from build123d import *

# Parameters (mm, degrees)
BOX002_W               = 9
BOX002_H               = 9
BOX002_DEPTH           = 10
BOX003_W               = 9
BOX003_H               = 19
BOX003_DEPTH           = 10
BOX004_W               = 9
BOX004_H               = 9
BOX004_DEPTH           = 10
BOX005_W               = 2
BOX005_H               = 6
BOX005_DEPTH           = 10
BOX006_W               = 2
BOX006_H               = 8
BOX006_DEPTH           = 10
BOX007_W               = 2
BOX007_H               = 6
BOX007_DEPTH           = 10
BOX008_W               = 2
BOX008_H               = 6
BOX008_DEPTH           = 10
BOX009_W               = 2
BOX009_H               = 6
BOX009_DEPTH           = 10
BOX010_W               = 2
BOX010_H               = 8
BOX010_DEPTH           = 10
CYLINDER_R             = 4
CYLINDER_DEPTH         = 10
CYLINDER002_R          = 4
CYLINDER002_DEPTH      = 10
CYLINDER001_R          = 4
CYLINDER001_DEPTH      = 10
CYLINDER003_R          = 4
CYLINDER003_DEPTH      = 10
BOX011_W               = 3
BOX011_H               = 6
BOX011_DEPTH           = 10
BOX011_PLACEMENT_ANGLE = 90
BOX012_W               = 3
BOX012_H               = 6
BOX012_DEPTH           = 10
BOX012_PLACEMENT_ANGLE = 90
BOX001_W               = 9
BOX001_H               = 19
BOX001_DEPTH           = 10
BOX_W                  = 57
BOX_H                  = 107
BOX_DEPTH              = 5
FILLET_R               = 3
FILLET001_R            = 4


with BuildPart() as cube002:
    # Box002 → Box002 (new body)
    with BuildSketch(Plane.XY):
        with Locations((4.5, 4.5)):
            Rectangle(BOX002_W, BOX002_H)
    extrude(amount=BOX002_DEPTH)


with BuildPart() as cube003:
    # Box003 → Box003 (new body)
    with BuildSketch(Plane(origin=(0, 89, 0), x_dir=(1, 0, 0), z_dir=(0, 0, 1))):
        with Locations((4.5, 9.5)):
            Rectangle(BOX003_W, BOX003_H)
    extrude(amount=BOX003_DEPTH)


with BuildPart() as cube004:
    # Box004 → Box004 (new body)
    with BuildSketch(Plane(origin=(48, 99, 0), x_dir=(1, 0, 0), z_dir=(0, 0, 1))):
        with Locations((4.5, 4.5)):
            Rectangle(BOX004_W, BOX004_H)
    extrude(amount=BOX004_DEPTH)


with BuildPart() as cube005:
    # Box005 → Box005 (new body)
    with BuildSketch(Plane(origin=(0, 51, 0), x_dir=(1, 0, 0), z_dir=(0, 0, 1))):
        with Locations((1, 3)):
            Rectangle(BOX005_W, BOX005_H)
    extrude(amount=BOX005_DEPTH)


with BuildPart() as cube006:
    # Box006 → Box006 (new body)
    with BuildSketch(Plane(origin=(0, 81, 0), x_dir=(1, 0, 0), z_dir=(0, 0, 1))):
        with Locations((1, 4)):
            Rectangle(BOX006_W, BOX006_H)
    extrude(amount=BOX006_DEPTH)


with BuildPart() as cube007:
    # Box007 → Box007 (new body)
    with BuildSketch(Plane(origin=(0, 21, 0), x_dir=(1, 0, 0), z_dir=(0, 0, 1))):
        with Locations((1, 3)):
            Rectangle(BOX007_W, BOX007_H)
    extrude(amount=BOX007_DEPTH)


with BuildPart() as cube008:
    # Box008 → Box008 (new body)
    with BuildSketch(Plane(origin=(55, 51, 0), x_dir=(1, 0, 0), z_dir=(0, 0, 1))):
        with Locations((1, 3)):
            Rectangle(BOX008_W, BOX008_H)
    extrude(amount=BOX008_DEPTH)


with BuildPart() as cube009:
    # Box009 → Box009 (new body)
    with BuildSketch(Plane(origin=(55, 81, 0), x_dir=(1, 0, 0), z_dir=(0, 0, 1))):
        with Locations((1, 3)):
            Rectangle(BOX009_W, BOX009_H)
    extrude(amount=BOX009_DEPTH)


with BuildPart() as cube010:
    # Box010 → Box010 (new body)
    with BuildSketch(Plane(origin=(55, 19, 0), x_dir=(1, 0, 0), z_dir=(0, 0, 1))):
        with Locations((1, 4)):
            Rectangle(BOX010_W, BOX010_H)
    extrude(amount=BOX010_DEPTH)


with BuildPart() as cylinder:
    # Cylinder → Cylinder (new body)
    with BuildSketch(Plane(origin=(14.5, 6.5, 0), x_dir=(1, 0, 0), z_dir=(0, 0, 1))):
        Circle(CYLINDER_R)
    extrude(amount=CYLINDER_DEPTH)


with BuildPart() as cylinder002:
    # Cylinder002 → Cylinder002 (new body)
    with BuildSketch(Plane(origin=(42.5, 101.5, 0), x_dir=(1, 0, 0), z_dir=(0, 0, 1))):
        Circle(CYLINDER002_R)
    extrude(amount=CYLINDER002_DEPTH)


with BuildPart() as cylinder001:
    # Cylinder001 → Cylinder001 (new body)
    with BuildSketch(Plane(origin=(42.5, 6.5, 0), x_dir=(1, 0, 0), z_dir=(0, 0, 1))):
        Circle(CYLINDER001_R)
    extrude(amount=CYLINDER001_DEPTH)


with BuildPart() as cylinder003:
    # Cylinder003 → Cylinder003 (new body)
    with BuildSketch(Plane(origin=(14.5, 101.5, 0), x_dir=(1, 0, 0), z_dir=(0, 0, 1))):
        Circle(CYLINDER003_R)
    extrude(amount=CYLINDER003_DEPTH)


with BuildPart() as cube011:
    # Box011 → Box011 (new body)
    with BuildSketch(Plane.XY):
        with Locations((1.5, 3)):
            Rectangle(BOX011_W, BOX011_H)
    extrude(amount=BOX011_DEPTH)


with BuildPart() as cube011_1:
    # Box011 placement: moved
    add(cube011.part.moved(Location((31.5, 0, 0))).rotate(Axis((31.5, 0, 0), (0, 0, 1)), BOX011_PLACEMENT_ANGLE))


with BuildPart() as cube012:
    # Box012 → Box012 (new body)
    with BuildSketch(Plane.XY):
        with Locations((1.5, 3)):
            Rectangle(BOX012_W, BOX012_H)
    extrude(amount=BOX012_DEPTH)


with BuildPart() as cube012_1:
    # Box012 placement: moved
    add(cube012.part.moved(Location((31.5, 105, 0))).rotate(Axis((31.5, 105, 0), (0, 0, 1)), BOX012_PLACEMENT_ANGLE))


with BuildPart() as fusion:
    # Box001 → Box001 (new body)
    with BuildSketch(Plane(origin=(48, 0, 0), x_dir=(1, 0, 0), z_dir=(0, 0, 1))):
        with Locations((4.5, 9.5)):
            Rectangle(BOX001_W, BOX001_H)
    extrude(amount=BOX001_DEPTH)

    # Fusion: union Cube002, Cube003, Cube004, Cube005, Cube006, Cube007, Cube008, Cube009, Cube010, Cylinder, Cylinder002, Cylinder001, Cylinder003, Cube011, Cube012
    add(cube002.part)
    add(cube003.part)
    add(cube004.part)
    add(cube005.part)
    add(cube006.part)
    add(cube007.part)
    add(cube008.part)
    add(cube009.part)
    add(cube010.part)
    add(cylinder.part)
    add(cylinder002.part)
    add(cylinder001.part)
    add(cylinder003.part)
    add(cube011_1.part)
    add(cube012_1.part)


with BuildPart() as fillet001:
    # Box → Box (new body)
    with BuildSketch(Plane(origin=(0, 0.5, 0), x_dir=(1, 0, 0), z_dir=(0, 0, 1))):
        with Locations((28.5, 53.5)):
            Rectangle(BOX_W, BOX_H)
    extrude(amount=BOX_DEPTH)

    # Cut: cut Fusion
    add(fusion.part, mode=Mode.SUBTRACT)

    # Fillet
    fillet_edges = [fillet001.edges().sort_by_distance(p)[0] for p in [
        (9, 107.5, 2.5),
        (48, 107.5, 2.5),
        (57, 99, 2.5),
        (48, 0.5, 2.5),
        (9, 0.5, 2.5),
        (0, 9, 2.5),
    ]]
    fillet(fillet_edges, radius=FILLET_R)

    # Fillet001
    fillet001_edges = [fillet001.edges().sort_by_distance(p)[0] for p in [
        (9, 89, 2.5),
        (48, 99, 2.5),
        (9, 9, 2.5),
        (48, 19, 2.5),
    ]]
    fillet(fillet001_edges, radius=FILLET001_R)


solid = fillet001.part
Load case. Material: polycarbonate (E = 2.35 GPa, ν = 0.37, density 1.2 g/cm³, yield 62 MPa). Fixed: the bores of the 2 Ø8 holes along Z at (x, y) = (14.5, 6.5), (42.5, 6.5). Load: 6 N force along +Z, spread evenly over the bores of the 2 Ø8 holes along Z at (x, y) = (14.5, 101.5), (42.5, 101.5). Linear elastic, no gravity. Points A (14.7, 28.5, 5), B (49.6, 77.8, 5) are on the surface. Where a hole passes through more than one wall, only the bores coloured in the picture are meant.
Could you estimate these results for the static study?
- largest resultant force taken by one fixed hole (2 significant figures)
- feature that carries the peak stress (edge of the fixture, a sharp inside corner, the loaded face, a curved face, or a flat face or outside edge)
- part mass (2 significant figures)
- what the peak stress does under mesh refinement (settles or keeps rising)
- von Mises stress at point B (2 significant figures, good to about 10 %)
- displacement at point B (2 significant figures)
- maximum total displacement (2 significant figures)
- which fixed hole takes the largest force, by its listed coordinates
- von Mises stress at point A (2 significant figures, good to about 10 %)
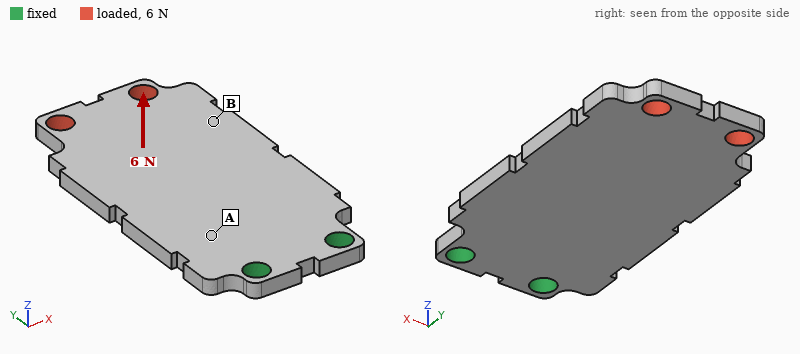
3.8 N
edge of the fixture
32 g
keeps rising
0.64 MPa
0.80 mm
1.4 mm
(14.5, 6.5)
1.9 MPa
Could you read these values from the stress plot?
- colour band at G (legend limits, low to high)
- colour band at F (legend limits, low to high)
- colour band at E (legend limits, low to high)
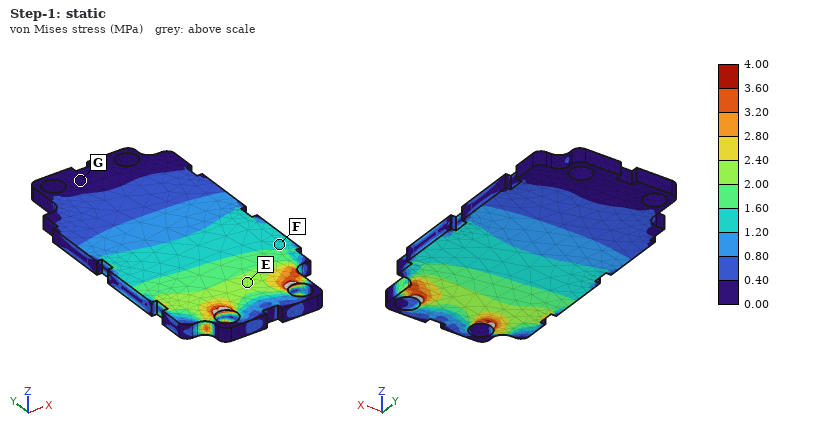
0.00 to 0.40 MPa
1.20 to 1.60 MPa
2.00 to 2.40 MPa
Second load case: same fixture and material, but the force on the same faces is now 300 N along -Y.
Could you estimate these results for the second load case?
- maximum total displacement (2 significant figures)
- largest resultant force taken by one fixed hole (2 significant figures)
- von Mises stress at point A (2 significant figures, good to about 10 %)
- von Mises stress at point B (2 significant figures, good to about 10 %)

83 µm
150 N
1.2 MPa
1.1 MPa
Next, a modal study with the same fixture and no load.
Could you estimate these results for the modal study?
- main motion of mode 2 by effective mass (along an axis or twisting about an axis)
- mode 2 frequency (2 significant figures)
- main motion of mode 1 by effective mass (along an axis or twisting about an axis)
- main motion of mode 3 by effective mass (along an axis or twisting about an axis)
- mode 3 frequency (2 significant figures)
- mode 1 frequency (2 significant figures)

twisting about Y
460 Hz
along Z
along Z
750 Hz
120 Hz
